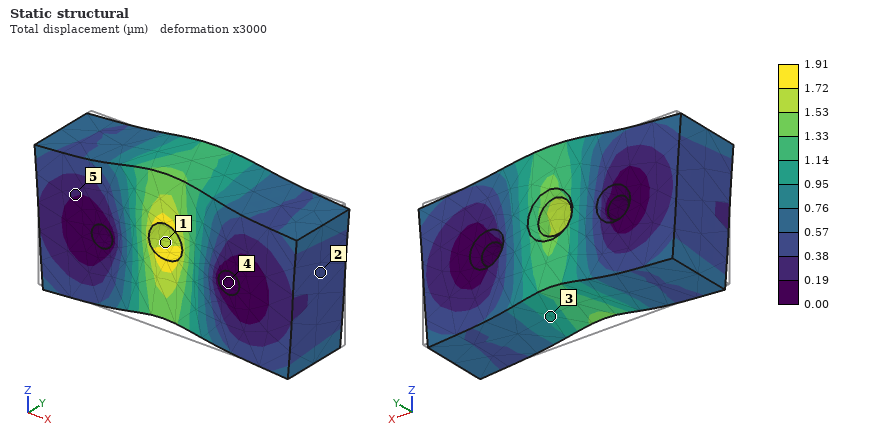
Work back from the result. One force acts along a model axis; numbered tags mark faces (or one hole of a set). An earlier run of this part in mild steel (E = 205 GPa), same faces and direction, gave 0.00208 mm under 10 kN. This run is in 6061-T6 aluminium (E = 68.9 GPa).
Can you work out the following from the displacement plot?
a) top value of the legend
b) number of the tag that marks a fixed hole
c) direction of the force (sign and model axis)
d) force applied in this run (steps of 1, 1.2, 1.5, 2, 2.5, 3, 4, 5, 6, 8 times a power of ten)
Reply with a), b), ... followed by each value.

a) 1.91 µm
b) 4
c) +Z
d) 3 kN
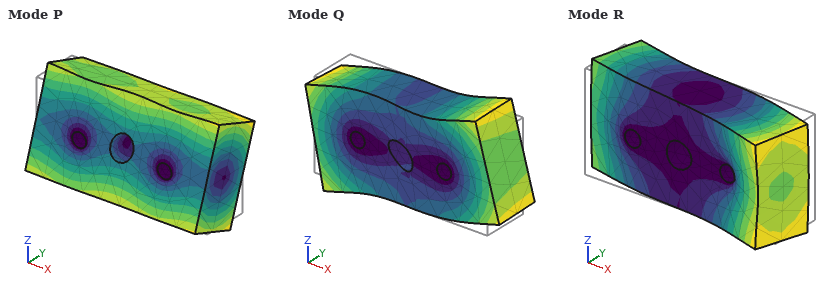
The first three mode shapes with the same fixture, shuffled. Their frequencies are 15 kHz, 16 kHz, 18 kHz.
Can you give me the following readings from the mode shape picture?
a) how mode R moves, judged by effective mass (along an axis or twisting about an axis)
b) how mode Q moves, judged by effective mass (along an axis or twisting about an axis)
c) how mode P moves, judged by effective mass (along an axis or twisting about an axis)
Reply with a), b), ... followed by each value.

a) twisting about Z
b) twisting about Y
c) twisting about X
